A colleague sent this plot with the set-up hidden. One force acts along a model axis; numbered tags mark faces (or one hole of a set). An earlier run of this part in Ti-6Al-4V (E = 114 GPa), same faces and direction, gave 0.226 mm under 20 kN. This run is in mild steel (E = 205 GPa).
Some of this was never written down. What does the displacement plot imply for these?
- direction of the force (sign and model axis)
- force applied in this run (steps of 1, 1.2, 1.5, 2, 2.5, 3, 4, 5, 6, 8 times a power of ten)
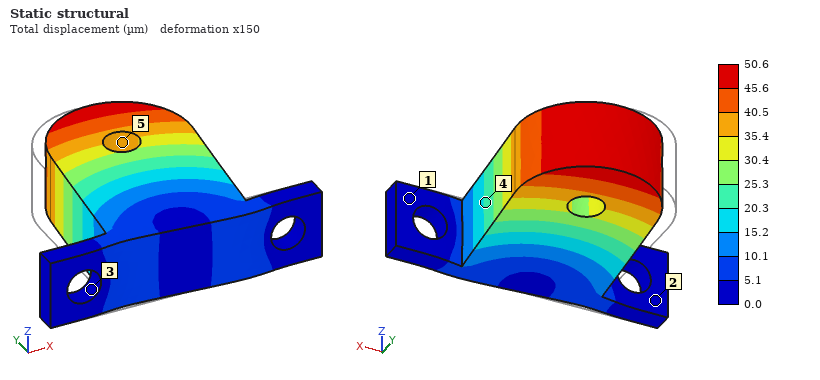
+X
8 kN
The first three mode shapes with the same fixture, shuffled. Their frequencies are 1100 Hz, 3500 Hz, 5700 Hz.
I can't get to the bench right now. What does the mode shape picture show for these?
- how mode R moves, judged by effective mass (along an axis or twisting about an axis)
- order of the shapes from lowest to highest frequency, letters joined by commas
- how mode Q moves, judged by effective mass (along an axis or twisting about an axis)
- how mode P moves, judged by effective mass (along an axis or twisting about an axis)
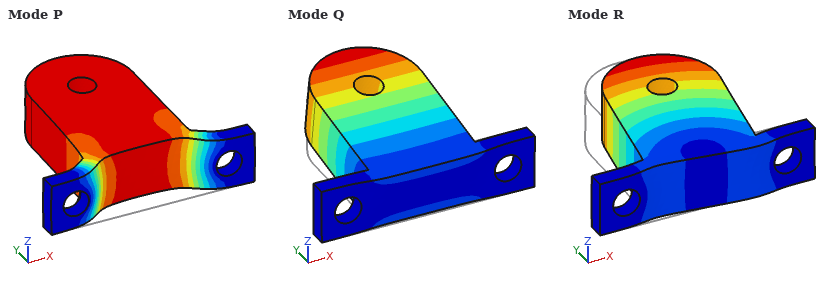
along X
Q, R, P
along Z
along Y
